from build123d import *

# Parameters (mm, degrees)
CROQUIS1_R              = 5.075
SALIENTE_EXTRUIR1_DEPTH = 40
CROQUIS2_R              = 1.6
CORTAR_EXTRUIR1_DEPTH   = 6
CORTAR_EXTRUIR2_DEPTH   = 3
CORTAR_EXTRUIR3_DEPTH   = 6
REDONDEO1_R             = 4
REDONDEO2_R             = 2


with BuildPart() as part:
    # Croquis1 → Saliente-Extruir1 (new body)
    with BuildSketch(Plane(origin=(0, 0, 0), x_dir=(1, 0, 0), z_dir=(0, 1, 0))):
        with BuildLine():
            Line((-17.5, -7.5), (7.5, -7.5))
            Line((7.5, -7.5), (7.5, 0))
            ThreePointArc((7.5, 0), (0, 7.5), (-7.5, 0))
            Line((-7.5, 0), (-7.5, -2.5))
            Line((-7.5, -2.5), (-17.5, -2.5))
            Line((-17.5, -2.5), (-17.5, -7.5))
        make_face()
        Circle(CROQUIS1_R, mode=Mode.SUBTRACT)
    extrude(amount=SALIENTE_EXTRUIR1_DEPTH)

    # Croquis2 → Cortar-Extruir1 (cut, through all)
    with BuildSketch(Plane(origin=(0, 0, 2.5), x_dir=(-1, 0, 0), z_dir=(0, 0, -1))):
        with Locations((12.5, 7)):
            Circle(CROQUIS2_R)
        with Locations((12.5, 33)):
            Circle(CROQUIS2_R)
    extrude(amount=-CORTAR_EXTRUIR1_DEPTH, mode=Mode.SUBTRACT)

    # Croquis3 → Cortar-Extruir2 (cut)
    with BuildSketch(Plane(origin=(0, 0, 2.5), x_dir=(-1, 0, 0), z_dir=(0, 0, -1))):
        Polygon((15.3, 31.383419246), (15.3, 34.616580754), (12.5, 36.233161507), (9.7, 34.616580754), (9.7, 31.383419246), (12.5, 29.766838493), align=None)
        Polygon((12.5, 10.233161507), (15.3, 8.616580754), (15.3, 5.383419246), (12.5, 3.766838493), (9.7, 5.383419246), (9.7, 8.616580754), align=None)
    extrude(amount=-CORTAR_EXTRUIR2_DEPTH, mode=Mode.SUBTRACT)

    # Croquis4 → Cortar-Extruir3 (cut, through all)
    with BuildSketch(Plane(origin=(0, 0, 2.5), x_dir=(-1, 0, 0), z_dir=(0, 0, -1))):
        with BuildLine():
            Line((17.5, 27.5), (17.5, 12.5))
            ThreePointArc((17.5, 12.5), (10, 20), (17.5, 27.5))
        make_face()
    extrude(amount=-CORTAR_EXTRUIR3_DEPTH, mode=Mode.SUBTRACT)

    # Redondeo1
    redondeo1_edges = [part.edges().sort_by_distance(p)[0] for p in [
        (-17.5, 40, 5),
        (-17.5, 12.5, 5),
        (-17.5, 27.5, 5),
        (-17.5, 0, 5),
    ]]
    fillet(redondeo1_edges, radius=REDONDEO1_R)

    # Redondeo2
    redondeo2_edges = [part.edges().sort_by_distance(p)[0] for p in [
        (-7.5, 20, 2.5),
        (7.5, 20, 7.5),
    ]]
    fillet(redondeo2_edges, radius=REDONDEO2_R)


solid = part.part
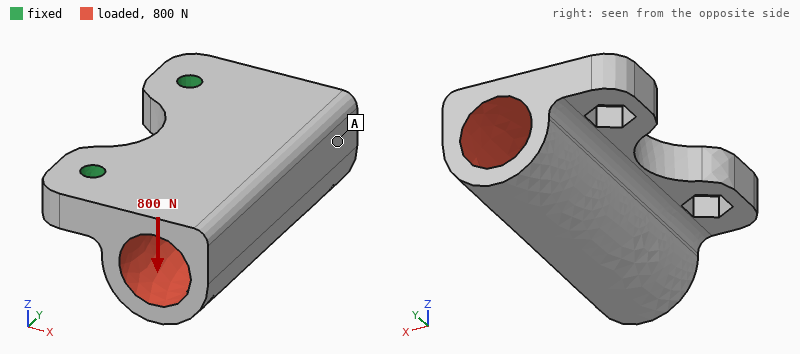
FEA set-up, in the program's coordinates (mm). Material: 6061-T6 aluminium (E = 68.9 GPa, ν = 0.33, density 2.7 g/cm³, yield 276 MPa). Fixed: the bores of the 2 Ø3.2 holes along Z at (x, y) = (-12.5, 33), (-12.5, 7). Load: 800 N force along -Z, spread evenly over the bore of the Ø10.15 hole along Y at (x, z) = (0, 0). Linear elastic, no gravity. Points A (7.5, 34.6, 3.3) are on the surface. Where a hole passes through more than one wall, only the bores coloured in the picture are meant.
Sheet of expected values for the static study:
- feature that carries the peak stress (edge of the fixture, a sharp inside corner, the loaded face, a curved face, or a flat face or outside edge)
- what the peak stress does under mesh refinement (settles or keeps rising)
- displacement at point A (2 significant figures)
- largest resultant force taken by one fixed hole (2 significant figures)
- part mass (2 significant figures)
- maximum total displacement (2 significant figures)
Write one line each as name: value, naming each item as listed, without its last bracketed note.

feature that carries the peak stress: edge of the fixture
what the peak stress does under mesh refinement: keeps rising
displacement at point A: 0.16 mm
largest resultant force taken by one fixed hole: 400 N
part mass: 16 g
maximum total displacement: 0.17 mm
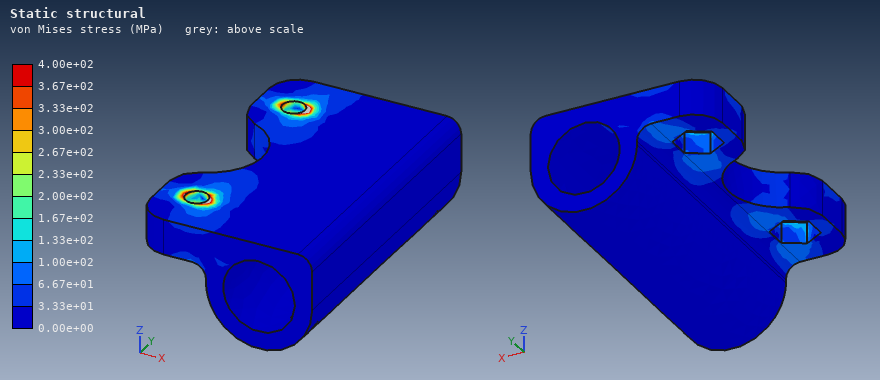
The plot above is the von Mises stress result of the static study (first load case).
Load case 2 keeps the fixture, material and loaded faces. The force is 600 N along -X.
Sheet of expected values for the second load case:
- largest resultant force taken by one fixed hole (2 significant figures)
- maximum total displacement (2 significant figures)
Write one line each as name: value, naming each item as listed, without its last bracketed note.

largest resultant force taken by one fixed hole: 310 N
maximum total displacement: 73 µm
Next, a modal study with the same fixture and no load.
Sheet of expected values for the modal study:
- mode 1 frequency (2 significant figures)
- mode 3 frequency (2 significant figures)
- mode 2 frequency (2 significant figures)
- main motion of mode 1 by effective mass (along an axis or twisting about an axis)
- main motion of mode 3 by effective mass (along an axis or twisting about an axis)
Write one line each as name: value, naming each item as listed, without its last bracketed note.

mode 1 frequency: 3300 Hz
mode 3 frequency: 16 kHz
mode 2 frequency: 13 kHz
main motion of mode 1 by effective mass: along Z
main motion of mode 3 by effective mass: along Y
